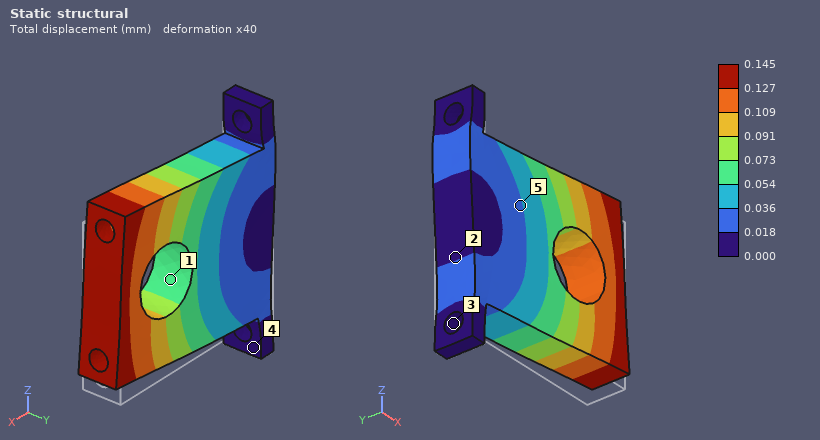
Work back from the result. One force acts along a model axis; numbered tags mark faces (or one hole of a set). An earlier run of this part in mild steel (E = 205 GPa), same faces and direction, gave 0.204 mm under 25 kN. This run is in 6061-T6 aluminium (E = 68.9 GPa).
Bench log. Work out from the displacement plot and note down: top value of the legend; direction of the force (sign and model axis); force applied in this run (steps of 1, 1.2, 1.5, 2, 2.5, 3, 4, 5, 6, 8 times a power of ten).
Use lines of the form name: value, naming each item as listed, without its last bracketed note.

top value of the legend: 0.145 mm
direction of the force: +Z
force applied in this run: 6 kN
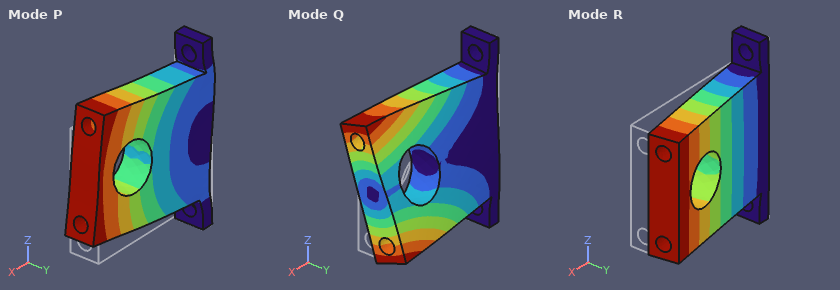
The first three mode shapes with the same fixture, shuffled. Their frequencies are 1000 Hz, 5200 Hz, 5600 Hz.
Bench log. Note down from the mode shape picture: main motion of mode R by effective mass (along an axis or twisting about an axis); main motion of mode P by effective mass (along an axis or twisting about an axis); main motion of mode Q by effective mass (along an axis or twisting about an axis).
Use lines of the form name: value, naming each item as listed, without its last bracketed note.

main motion of mode R by effective mass: along Y
main motion of mode P by effective mass: along Z
main motion of mode Q by effective mass: twisting about X
